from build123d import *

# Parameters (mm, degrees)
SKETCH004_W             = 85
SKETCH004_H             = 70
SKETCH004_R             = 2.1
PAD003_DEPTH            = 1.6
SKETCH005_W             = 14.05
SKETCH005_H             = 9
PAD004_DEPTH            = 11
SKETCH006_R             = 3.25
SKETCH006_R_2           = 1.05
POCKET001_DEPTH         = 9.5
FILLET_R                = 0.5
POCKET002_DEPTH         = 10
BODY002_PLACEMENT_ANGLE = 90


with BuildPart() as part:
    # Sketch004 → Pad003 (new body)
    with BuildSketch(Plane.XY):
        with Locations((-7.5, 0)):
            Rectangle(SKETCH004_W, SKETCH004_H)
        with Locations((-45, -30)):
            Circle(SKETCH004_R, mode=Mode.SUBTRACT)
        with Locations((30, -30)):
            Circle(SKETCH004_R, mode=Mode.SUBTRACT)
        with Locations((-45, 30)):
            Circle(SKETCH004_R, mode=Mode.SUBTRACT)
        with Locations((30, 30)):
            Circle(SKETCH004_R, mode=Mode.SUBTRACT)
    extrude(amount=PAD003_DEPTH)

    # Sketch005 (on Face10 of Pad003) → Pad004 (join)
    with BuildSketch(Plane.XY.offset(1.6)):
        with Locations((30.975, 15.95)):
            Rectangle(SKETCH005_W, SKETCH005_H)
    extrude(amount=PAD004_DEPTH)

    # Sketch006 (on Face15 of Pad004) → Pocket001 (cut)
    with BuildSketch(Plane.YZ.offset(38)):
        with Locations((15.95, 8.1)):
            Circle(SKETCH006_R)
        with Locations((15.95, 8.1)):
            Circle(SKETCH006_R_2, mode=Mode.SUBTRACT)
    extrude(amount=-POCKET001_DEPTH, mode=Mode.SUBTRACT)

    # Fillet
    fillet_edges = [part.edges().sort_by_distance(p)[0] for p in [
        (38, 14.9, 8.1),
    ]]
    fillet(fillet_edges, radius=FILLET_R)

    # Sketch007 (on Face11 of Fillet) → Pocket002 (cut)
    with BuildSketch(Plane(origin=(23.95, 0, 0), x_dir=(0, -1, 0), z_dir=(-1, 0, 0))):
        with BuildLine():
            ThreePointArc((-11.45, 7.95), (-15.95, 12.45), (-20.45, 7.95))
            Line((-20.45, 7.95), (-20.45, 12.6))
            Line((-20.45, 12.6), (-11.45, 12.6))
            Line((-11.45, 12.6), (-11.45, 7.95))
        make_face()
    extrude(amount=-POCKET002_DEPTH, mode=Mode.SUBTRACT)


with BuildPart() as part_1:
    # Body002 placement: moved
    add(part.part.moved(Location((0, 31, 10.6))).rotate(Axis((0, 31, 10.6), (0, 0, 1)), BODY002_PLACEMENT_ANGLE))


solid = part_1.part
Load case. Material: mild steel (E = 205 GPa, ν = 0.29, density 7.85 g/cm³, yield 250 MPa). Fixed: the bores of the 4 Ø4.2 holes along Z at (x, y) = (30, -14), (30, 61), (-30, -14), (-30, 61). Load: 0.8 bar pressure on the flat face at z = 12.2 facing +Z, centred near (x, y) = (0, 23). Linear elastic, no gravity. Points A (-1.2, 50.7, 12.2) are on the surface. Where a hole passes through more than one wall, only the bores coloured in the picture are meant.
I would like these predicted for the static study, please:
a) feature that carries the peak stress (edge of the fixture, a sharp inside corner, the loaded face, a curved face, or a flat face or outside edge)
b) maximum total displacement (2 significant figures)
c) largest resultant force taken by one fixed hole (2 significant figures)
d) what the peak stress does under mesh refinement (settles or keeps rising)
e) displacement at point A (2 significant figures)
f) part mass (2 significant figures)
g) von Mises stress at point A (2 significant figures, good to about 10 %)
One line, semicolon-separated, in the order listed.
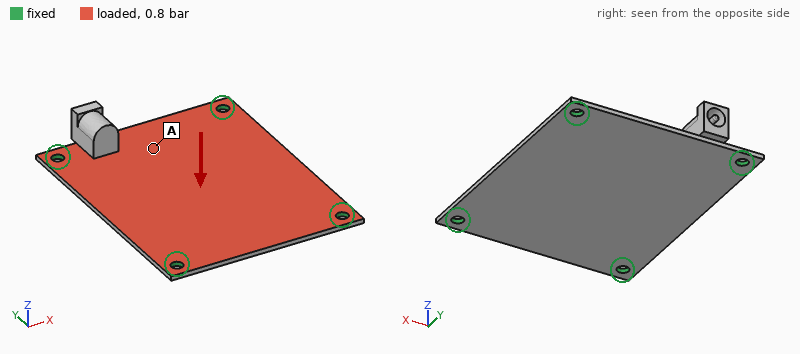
edge of the fixture; 0.16 mm; 120 N; keeps rising; 0.089 mm; 82 g; 37 MPa
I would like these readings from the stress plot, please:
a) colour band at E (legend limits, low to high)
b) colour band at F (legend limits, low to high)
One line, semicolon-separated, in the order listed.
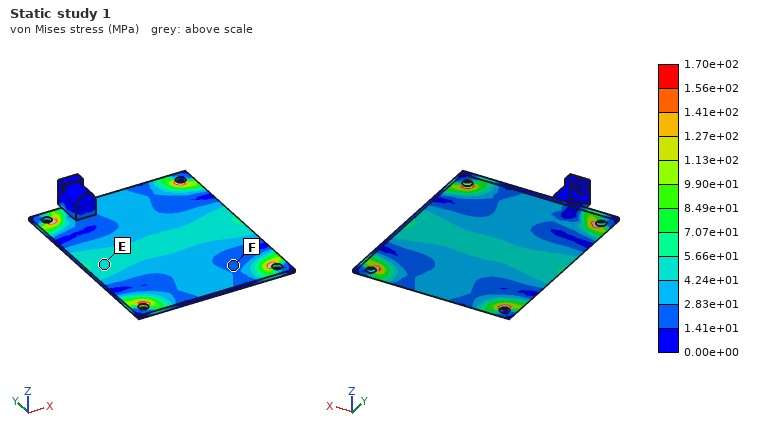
4.24e+01 to 5.66e+01 MPa; 1.41e+01 to 2.83e+01 MPa
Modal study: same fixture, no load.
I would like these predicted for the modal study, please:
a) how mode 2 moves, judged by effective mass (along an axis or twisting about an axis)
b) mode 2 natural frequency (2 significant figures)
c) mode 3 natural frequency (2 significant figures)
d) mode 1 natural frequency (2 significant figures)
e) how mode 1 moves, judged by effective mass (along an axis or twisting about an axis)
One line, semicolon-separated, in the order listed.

twisting about Y; 1900 Hz; 2200 Hz; 1200 Hz; along Z
